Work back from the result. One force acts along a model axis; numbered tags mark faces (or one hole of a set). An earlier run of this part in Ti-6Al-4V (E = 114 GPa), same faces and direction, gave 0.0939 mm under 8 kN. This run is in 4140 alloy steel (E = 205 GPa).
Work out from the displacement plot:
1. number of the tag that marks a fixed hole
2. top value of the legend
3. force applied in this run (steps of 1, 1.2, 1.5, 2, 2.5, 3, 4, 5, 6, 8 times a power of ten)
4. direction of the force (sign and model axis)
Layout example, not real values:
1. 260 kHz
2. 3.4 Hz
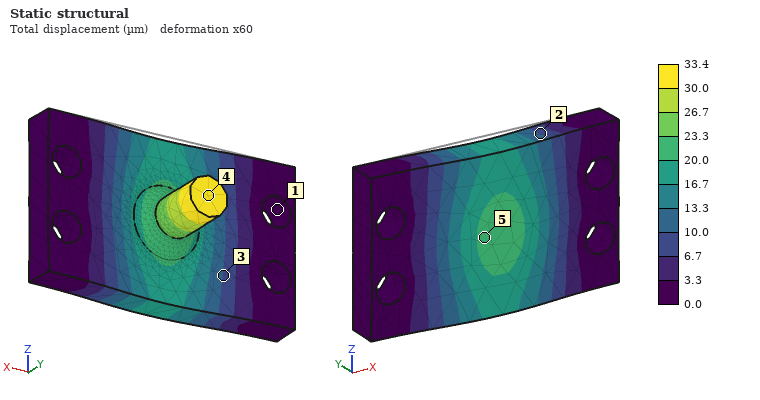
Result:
1. 1
2. 33.4 µm
3. 5 kN
4. -Y
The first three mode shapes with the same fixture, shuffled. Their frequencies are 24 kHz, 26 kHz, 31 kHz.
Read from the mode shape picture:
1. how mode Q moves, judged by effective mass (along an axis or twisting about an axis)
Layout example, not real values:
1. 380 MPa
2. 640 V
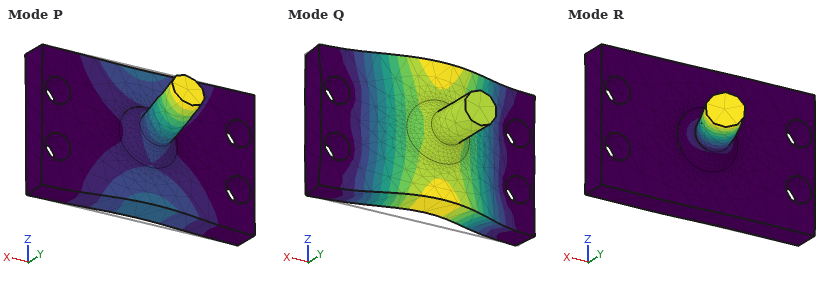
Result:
1. along Y
